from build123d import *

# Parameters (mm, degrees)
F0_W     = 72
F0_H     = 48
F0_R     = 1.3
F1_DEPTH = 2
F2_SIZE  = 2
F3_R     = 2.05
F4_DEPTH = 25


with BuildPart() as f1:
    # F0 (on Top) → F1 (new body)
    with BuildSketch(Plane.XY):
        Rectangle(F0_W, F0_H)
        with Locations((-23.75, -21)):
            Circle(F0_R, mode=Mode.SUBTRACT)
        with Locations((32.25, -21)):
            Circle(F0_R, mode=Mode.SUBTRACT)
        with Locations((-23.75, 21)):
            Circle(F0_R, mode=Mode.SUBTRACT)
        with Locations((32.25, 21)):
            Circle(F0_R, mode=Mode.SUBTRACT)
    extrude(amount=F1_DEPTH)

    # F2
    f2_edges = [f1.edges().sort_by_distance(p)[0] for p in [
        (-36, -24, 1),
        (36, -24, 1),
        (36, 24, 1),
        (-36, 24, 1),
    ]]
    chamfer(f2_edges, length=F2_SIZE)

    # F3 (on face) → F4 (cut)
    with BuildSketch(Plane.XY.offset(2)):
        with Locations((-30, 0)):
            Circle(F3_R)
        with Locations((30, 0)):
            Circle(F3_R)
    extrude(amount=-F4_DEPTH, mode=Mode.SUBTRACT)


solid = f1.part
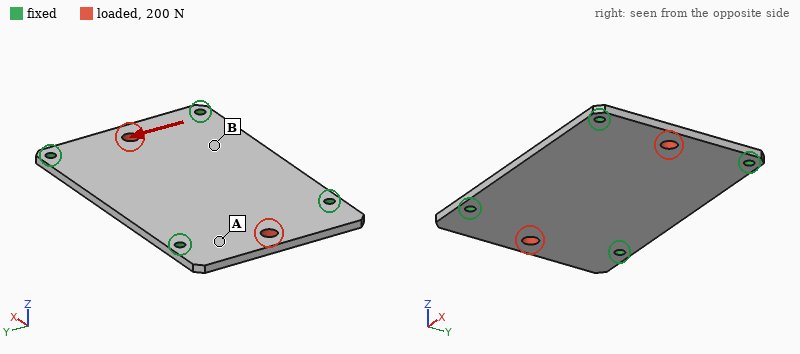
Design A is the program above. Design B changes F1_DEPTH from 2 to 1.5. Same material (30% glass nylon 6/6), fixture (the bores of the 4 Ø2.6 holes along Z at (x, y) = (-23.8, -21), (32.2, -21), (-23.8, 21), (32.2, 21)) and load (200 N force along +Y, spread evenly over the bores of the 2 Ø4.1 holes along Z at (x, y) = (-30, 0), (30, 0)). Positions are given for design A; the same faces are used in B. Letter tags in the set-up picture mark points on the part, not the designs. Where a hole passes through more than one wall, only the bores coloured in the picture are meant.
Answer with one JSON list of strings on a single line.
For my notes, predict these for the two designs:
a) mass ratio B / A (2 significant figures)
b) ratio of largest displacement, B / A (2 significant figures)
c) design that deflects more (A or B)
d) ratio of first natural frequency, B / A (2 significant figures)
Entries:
["0.75", "1.3", "B", "0.76"]
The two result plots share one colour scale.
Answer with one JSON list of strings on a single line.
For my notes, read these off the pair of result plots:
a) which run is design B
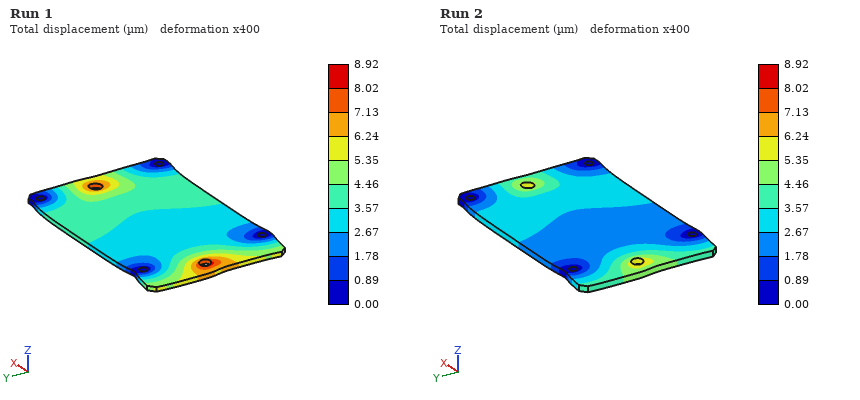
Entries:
["Run 1"]
